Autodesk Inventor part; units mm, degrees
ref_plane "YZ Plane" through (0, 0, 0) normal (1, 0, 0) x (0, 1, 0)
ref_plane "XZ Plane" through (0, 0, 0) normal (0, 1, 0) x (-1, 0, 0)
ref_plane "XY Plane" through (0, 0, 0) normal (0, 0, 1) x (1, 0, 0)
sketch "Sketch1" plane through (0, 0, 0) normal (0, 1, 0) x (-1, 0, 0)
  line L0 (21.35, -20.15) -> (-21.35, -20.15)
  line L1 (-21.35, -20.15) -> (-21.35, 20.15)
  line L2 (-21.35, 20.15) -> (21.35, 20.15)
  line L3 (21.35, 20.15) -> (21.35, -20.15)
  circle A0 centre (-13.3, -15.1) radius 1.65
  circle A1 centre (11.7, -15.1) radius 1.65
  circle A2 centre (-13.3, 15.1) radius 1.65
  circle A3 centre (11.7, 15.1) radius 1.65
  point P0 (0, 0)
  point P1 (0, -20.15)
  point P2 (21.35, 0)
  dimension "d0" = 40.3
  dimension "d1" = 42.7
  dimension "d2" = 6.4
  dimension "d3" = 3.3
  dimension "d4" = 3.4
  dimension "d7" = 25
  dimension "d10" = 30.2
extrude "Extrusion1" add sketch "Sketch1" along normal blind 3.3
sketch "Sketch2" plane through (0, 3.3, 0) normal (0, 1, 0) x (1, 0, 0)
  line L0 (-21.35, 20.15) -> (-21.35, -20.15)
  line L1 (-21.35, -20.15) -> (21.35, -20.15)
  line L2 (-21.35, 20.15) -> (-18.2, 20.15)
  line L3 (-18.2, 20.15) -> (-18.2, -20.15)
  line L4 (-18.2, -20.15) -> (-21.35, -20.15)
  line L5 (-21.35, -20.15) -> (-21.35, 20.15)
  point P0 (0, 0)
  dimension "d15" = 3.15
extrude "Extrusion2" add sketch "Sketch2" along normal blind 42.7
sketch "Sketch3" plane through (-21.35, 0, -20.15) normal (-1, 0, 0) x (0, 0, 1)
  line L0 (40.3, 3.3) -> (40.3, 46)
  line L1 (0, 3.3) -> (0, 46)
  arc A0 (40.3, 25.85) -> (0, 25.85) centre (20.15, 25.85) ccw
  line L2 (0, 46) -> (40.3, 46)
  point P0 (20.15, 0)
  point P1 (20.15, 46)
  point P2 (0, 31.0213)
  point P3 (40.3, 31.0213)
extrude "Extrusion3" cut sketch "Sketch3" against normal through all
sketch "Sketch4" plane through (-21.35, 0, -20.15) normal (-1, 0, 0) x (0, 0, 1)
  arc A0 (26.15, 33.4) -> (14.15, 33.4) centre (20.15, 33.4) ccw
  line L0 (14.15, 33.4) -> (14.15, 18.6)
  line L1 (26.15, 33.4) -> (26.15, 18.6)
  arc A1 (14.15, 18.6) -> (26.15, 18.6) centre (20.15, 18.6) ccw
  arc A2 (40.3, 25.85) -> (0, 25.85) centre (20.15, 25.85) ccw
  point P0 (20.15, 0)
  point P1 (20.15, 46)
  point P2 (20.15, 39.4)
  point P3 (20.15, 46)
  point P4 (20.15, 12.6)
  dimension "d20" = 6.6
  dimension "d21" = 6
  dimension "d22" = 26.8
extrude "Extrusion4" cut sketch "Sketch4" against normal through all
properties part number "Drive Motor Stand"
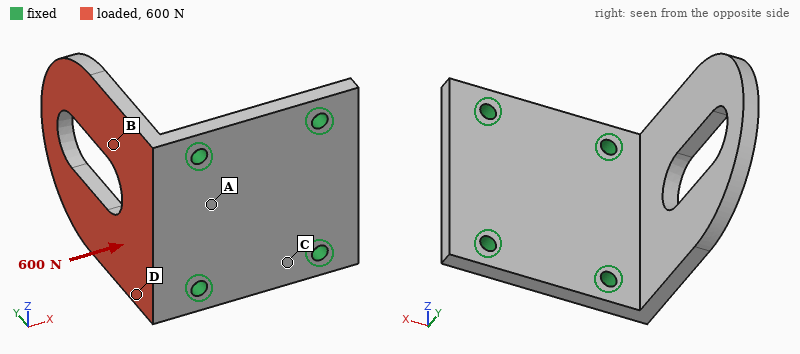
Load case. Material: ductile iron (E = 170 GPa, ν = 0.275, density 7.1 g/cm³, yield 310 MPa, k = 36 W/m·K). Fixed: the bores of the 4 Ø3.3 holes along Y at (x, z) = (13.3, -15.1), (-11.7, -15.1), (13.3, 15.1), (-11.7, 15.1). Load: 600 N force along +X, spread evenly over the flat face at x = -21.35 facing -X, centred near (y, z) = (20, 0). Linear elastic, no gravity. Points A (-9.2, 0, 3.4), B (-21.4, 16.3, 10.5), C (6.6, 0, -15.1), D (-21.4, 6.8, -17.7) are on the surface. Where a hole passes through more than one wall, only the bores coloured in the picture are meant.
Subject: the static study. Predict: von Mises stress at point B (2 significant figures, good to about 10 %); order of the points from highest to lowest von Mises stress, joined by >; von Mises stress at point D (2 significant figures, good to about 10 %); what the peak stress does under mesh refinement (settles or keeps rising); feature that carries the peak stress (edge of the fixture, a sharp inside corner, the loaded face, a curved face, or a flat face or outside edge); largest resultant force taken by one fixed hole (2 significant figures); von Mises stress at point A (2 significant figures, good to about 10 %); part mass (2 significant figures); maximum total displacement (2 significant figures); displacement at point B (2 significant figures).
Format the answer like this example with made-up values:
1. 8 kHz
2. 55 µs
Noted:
1. 93 MPa
2. D > B > A > C
3. 130 MPa
4. keeps rising
5. edge of the fixture
6. 230 N
7. 50 MPa
8. 68 g
9. 0.50 mm
10. 0.12 mm
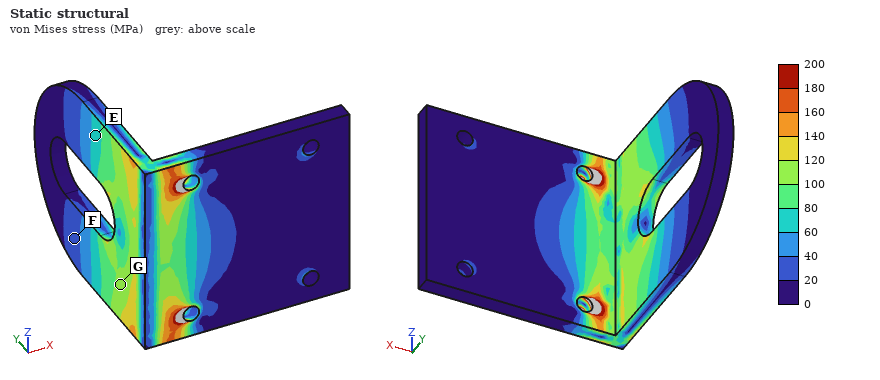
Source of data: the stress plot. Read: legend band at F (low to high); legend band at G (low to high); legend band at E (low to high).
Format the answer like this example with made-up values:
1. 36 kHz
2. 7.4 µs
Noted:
1. 20 to 40 MPa
2. 100 to 120 MPa
3. 60 to 80 MPa
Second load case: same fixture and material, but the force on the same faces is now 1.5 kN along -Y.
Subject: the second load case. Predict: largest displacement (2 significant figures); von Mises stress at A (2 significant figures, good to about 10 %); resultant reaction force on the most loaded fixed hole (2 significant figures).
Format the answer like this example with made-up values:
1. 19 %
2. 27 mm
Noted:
1. 0.25 mm
2. 48 MPa
3. 820 N
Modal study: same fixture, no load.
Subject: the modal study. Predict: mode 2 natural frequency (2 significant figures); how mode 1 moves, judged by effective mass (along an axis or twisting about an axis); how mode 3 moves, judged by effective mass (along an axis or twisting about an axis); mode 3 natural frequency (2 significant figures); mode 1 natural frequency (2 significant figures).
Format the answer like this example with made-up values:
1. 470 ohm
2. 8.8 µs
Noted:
1. 3400 Hz
2. along X
3. along Z
4. 5500 Hz
5. 1300 Hz
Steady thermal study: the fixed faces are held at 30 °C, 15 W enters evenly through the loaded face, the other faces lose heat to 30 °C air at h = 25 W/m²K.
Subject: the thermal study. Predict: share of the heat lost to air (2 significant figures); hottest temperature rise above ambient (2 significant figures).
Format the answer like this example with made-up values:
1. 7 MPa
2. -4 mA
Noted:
1. 22 %
2. 82 K
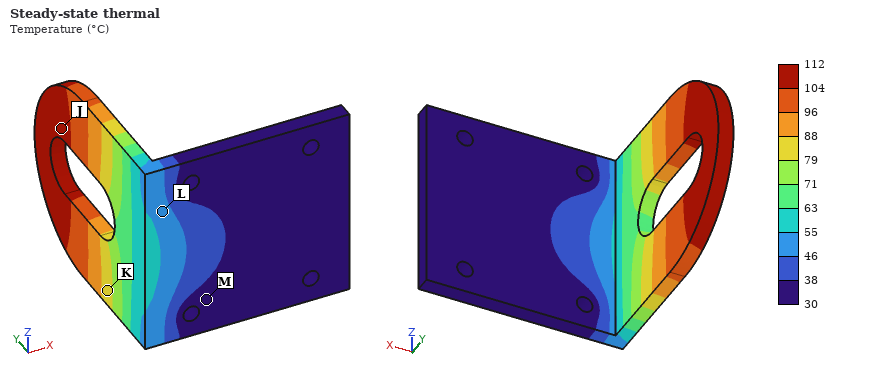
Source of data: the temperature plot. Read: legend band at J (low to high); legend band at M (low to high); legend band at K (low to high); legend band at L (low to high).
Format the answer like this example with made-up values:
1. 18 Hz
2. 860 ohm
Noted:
1. 104 to 112 °C
2. 30 to 38 °C
3. 79 to 88 °C
4. 46 to 55 °C
